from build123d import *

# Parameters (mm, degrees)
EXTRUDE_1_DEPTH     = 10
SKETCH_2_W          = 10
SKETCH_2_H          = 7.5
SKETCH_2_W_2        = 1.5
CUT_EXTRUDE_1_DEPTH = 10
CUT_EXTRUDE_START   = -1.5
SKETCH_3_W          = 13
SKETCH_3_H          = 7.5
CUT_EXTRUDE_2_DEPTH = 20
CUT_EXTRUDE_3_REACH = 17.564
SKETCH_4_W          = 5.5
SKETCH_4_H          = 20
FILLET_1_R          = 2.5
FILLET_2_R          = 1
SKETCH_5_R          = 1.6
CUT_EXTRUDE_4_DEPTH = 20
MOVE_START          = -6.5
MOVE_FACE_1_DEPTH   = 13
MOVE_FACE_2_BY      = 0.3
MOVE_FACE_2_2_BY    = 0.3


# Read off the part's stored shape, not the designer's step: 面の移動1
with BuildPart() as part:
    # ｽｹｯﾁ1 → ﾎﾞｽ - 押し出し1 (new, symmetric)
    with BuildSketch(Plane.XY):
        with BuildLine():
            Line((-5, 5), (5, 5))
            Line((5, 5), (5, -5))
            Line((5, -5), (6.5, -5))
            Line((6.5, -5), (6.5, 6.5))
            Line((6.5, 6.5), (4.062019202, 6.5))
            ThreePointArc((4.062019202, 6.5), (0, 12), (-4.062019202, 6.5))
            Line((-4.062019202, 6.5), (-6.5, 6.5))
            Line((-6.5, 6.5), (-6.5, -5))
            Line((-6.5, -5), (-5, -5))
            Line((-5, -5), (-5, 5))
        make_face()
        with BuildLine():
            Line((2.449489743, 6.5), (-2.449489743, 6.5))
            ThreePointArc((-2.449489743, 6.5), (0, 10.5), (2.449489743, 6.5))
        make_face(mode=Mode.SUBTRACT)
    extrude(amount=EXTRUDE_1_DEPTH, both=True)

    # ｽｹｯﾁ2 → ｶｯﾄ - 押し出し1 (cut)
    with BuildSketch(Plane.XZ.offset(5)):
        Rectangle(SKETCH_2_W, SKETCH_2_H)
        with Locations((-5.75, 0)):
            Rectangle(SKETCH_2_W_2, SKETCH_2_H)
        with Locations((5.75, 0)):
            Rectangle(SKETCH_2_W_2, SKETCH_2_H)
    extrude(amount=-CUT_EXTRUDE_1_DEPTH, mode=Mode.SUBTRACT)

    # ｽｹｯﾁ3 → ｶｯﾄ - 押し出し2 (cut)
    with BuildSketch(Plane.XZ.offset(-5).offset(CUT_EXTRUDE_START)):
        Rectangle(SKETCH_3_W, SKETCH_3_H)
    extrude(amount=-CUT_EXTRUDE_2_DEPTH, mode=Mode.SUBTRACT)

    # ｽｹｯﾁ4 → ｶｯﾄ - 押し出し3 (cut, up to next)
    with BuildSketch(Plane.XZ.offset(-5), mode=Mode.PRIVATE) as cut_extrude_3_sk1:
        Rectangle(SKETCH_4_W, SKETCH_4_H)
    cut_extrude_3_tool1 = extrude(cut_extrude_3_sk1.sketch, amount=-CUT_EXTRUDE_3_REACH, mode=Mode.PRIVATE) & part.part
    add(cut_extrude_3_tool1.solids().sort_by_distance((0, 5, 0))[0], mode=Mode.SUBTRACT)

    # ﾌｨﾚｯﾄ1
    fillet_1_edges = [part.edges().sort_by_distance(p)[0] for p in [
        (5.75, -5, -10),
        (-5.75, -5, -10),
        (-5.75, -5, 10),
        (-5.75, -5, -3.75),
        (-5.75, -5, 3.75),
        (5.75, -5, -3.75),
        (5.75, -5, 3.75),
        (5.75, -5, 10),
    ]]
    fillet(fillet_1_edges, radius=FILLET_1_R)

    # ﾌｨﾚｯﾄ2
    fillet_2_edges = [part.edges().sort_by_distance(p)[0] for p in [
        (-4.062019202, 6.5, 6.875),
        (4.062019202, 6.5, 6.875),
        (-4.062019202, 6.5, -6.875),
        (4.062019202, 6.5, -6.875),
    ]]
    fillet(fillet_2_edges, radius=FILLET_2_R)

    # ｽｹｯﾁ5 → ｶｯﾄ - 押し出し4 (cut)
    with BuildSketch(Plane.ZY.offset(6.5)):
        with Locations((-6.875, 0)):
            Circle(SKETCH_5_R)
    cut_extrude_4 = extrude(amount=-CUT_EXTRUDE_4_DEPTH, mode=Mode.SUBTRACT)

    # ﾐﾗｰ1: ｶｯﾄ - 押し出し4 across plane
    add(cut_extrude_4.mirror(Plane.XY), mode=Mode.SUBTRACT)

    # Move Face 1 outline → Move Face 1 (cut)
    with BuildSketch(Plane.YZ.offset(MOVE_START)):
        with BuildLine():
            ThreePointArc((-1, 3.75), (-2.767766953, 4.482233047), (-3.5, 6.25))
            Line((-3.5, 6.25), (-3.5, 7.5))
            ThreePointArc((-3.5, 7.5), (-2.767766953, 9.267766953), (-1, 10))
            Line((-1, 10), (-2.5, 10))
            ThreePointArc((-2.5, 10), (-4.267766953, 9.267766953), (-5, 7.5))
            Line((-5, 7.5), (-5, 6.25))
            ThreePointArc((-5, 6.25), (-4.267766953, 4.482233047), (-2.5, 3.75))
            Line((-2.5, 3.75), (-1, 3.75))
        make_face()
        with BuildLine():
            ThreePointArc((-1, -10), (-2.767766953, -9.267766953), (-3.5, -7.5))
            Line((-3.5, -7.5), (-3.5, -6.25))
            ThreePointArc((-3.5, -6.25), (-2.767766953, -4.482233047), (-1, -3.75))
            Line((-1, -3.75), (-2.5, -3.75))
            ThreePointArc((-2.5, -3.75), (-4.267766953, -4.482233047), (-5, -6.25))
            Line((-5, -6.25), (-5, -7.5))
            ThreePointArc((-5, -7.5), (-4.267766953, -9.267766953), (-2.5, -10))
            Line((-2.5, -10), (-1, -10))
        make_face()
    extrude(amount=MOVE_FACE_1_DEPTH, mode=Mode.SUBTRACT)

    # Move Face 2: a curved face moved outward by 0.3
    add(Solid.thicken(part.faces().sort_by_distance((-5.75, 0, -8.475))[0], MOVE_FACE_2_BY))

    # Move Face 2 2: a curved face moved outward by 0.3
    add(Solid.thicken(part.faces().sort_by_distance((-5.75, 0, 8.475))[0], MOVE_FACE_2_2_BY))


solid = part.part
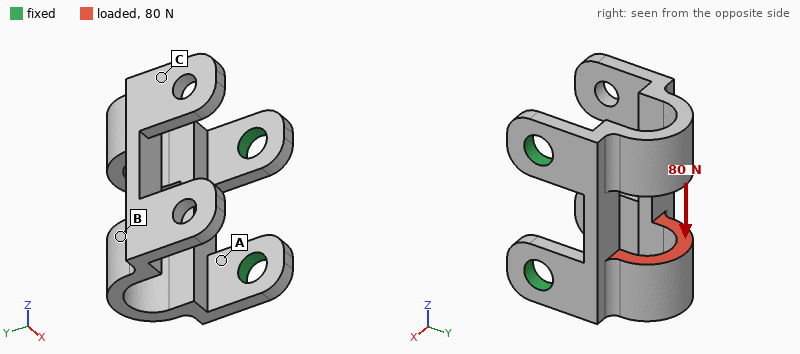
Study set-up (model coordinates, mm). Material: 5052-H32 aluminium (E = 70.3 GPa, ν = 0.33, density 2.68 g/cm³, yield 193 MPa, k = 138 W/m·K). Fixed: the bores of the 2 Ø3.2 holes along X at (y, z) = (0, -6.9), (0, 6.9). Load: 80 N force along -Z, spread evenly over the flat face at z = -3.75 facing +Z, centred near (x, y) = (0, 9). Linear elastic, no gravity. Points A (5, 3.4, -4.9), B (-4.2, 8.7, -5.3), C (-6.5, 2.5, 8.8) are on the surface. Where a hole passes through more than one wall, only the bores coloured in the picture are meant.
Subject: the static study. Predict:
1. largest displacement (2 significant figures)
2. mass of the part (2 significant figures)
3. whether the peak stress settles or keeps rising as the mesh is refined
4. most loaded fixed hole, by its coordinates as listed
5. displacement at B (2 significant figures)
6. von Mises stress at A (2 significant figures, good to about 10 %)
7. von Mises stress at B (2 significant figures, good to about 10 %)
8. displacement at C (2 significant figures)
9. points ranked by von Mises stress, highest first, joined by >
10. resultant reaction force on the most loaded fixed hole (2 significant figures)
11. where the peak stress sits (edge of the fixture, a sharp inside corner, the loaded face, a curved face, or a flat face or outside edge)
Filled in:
58 µm
2.0 g
keeps rising
(0, 6.9)
34 µm
38 MPa
16 MPa
47 µm
A > B > C
62 N
edge of the fixture
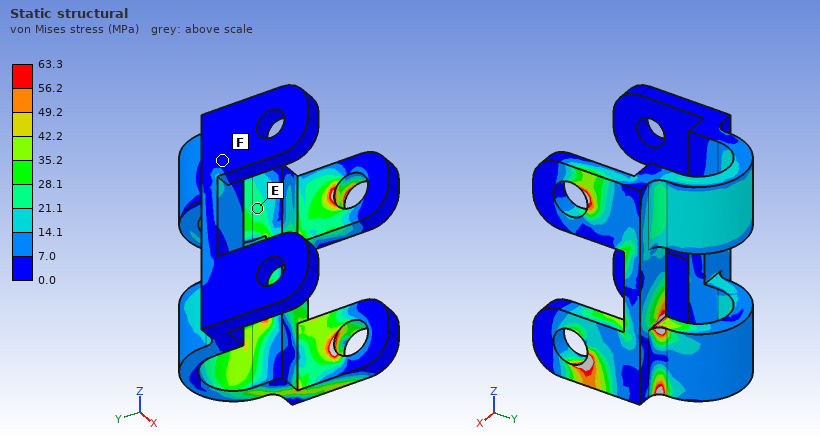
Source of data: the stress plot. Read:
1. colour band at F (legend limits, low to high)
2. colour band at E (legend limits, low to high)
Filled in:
0.0 to 7.0 MPa
21.1 to 28.1 MPa
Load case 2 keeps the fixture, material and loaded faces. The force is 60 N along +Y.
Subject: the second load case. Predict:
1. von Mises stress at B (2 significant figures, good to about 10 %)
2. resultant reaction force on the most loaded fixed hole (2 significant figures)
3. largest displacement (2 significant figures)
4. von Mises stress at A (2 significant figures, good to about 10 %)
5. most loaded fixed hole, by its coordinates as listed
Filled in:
7.1 MPa
49 N
0.18 mm
90 MPa
(0, -6.9)
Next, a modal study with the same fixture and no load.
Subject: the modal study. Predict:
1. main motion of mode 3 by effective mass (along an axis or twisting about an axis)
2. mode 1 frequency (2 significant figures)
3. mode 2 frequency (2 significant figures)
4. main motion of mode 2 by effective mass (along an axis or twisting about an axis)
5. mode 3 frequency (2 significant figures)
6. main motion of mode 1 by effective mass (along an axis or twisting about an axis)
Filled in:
along X
2200 Hz
3600 Hz
along Z
4500 Hz
along Y
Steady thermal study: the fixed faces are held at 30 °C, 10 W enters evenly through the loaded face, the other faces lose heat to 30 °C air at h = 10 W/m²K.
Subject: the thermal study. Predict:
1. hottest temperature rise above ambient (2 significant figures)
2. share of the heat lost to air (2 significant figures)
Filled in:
68 K
4.0 %
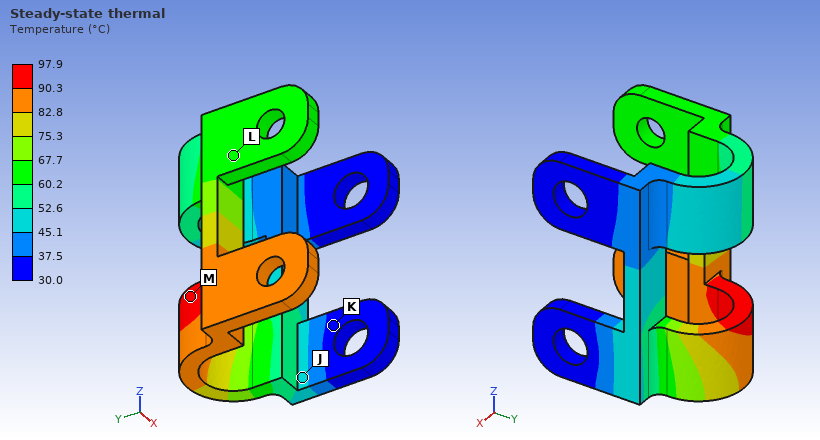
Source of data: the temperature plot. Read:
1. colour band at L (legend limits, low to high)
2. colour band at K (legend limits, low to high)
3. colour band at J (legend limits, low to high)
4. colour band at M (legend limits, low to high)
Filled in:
60.2 to 67.7 °C
30.0 to 37.5 °C
45.1 to 52.6 °C
90.3 to 97.9 °C
